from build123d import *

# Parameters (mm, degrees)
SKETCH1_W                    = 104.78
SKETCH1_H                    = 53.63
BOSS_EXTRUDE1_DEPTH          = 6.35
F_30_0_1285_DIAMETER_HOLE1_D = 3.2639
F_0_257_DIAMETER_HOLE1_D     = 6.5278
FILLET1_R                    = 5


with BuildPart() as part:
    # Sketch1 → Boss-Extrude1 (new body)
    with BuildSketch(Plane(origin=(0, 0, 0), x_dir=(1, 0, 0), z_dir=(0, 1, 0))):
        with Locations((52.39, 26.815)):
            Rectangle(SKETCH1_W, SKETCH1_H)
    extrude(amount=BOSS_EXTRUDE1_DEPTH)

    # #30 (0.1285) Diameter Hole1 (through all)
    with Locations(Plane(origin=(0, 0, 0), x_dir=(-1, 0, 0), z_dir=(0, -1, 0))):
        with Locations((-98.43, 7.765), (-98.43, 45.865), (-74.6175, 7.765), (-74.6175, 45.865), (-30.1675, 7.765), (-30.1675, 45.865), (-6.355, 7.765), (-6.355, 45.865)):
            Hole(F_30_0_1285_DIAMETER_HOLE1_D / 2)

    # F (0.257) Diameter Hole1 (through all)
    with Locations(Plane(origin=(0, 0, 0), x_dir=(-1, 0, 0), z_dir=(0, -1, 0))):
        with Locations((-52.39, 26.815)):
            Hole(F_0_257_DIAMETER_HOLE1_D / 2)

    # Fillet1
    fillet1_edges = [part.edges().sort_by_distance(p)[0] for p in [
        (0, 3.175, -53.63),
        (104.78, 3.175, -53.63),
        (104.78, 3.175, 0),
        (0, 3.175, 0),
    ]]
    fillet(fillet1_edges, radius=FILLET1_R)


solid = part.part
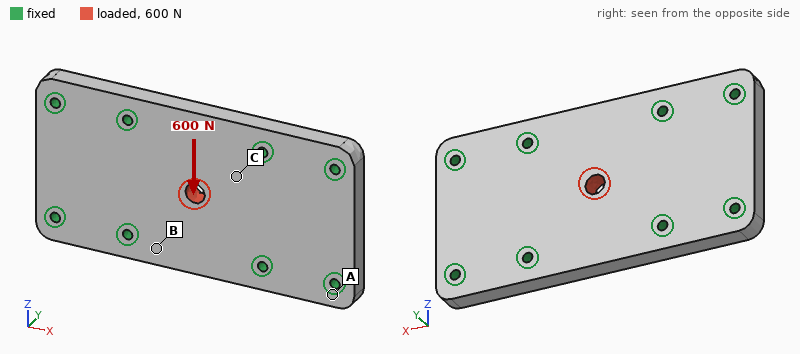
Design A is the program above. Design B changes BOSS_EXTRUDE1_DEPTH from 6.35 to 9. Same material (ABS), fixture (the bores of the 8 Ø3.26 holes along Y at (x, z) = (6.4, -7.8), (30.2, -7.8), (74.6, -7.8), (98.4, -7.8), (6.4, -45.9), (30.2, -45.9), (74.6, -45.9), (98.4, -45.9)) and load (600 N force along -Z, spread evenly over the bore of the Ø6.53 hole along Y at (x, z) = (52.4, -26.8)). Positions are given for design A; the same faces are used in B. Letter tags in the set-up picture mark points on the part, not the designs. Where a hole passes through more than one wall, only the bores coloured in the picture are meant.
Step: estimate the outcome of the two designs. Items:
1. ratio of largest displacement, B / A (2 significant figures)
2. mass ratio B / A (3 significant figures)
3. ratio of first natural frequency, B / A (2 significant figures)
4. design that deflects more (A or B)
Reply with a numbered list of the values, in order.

1. 0.70
2. 1.42
3. 1.3
4. A
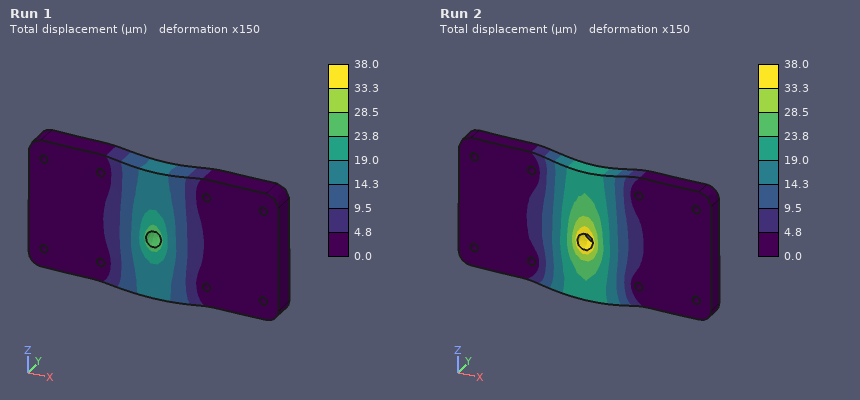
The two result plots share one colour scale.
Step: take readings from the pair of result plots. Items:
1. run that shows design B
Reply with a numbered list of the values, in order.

1. Run 1
